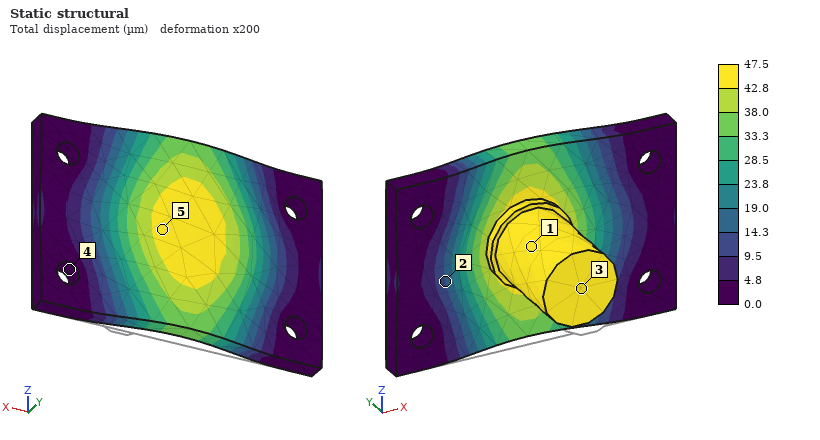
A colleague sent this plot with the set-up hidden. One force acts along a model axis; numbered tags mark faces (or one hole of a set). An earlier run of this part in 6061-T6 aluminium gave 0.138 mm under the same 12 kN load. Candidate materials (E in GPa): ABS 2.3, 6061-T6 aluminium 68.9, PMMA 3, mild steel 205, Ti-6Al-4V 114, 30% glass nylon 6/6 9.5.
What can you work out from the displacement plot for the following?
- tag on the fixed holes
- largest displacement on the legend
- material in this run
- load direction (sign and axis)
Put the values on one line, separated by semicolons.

4; 47.5 µm; mild steel; +Y
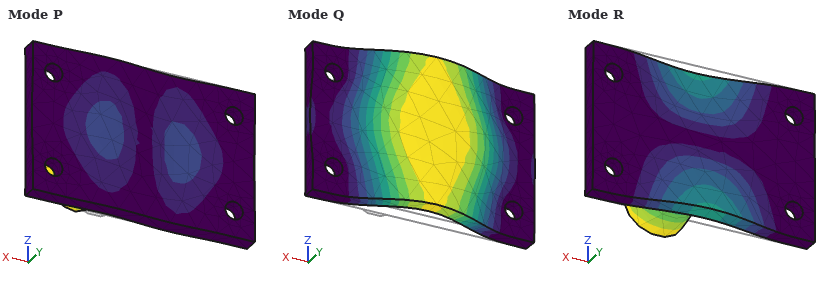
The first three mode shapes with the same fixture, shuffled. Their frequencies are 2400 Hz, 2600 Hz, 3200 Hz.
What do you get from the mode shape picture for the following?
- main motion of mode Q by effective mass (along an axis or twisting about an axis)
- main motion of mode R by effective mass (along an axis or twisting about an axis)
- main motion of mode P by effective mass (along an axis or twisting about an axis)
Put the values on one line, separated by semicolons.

along Y; along Z; along X
